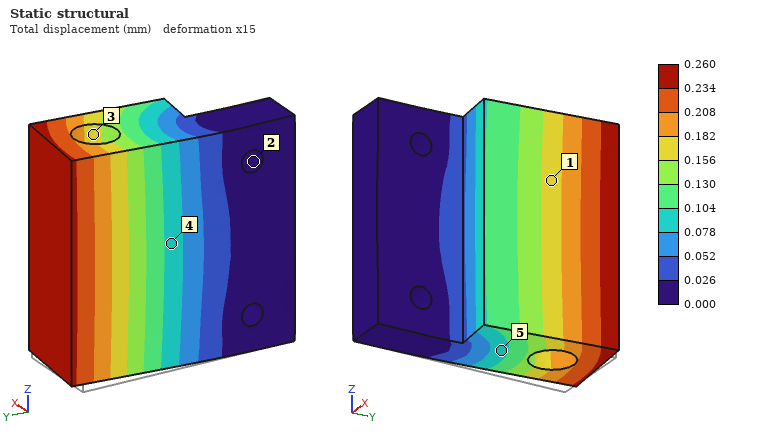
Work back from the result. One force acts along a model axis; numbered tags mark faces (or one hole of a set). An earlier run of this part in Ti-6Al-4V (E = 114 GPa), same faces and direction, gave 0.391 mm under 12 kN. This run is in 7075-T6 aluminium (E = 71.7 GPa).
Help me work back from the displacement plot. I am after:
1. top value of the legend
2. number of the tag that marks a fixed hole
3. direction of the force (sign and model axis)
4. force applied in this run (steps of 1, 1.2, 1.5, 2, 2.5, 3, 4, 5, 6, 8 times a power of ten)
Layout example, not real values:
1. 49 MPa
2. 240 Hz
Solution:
1. 0.260 mm
2. 2
3. +X
4. 5 kN
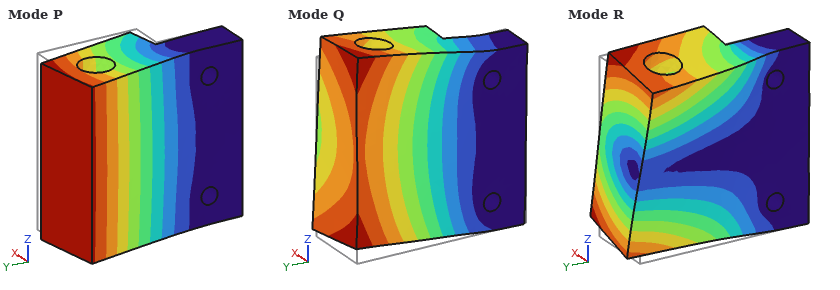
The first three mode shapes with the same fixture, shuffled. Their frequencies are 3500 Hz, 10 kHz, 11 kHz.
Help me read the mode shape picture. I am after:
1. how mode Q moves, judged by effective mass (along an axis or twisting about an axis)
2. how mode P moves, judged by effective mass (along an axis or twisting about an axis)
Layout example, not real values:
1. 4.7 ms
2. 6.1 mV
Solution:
1. along Z
2. along X
